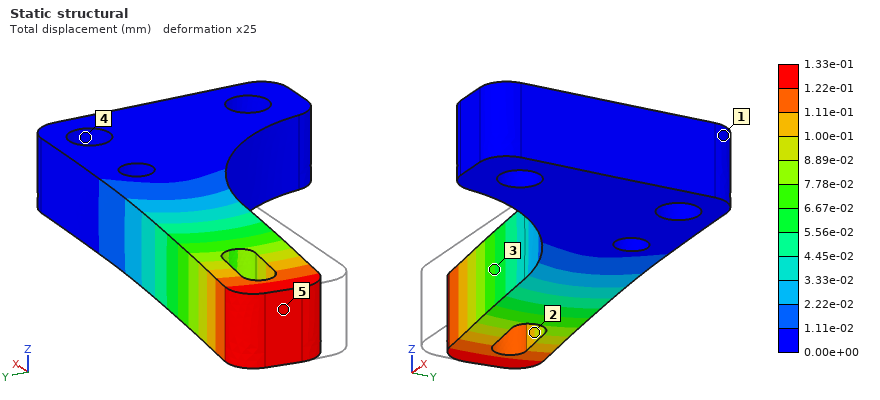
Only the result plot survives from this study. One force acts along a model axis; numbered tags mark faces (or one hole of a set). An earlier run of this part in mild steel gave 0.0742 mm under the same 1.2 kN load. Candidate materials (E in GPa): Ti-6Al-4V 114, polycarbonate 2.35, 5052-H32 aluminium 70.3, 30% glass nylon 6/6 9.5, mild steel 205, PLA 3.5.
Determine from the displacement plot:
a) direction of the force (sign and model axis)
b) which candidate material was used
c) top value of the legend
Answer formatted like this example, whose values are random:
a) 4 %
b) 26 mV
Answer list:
a) +Y
b) Ti-6Al-4V
c) 1.33e-01 mm
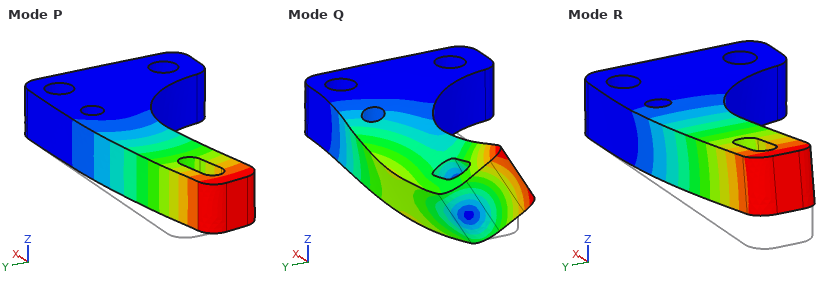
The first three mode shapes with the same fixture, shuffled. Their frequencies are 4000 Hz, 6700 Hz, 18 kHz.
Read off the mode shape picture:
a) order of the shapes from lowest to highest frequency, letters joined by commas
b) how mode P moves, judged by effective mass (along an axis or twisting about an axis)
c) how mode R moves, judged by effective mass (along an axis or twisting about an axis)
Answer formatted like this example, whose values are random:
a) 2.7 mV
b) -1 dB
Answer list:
a) R, P, Q
b) along Y
c) along Z
